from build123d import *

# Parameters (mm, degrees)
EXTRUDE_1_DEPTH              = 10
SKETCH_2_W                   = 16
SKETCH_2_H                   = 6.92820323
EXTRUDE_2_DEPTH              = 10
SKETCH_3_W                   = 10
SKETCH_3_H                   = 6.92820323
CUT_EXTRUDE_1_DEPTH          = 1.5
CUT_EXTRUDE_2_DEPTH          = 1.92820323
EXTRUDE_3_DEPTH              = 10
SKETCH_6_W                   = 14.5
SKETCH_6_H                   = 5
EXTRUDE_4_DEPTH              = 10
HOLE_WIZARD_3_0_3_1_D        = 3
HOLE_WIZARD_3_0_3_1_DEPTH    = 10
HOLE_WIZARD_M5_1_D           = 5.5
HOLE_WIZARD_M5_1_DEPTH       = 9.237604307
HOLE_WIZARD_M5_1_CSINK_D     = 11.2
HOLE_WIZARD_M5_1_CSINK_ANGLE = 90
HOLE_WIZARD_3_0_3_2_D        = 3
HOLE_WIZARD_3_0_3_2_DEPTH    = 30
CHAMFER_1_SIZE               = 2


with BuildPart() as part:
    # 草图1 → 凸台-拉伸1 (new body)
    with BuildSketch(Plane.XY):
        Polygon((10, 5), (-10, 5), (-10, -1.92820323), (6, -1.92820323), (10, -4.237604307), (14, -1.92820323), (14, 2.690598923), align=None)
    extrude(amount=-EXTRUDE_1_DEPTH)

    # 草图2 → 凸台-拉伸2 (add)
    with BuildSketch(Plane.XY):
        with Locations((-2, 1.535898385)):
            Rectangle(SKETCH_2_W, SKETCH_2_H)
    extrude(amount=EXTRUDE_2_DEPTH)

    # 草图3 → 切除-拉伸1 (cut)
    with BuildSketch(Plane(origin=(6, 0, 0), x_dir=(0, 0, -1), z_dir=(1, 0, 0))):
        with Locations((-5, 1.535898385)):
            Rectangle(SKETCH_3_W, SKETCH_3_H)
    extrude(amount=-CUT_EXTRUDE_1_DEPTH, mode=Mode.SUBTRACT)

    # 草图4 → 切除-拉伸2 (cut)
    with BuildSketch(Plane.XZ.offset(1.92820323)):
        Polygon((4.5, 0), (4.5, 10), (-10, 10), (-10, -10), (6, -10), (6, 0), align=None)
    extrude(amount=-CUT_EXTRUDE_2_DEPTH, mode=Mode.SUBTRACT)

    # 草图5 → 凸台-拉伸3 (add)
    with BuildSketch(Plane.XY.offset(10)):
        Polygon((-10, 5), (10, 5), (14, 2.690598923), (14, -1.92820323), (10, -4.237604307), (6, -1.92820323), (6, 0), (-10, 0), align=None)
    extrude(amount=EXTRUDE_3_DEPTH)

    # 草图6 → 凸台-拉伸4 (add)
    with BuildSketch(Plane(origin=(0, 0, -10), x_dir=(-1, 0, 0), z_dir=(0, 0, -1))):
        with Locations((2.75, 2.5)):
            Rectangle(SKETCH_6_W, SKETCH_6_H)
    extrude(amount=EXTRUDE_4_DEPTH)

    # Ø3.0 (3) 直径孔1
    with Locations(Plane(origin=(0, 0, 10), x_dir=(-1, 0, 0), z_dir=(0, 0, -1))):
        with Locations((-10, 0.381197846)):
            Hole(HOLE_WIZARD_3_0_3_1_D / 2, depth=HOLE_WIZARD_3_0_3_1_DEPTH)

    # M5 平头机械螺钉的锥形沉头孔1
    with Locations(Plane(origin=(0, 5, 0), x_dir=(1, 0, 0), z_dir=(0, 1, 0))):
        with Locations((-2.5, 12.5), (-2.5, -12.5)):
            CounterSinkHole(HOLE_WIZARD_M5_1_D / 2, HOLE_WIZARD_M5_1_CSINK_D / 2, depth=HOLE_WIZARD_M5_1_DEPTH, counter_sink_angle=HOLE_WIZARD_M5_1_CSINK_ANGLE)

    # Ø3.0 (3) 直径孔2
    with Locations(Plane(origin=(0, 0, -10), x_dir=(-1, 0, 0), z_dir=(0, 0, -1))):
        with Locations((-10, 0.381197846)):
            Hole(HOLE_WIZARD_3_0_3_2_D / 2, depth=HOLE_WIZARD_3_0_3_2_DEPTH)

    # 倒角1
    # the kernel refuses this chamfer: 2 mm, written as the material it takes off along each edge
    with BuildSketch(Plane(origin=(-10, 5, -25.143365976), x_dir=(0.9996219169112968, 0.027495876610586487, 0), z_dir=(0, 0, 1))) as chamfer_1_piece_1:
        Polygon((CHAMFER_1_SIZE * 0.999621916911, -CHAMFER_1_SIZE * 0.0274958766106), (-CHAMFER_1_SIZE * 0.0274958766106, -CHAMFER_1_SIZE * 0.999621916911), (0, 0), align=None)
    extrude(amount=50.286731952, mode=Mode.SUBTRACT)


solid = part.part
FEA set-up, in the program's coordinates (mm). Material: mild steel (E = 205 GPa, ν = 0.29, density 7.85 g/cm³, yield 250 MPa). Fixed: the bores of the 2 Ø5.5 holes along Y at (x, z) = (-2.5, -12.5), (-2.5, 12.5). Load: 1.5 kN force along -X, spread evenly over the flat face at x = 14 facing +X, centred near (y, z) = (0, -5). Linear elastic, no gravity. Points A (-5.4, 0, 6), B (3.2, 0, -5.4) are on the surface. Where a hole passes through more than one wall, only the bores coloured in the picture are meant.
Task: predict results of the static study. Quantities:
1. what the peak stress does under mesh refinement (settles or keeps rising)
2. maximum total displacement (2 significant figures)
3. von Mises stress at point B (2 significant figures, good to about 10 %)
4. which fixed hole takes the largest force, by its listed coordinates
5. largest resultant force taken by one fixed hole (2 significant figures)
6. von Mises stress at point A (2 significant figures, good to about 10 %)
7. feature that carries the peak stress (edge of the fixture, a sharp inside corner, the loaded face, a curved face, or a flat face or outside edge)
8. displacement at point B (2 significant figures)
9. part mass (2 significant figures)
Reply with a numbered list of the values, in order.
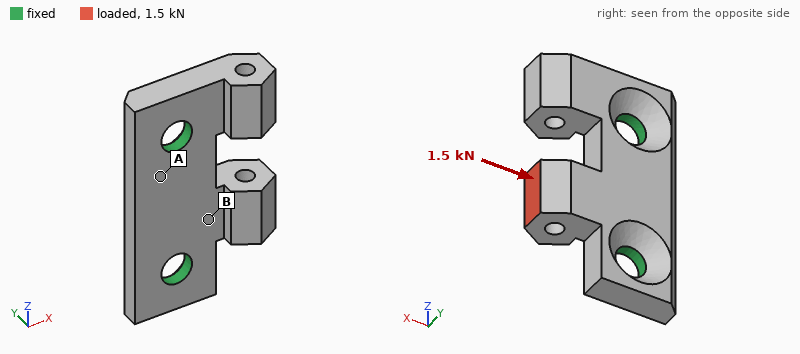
1. keeps rising
2. 19 µm
3. 75 MPa
4. (-2.5, -12.5)
5. 1.1 kN
6. 23 MPa
7. a sharp inside corner
8. 3.9 µm
9. 28 g
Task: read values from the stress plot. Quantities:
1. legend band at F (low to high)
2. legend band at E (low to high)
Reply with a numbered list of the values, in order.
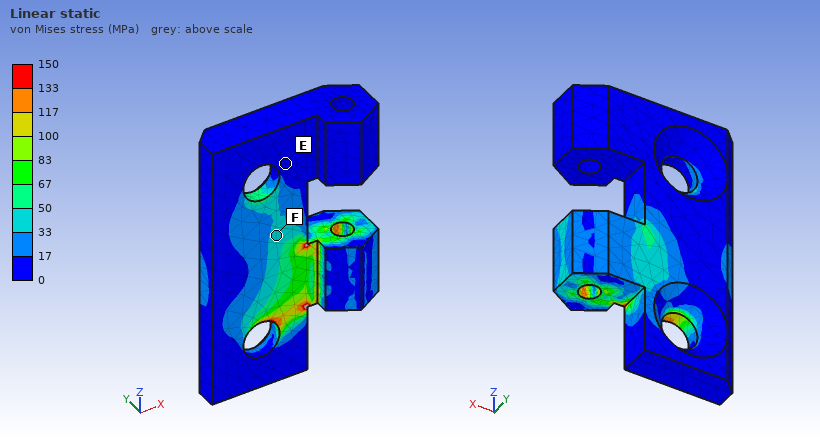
1. 33 to 50 MPa
2. 0 to 17 MPa
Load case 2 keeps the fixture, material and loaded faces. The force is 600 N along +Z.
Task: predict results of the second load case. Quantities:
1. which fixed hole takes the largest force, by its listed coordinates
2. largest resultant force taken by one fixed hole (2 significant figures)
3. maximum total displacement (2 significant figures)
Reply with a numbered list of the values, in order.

1. (-2.5, -12.5)
2. 560 N
3. 11 µm
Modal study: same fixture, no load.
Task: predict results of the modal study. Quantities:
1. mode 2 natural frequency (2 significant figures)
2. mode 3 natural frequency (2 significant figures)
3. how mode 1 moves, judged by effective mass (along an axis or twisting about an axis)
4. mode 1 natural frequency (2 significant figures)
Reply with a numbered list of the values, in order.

1. 12 kHz
2. 21 kHz
3. along Y
4. 10 kHz
